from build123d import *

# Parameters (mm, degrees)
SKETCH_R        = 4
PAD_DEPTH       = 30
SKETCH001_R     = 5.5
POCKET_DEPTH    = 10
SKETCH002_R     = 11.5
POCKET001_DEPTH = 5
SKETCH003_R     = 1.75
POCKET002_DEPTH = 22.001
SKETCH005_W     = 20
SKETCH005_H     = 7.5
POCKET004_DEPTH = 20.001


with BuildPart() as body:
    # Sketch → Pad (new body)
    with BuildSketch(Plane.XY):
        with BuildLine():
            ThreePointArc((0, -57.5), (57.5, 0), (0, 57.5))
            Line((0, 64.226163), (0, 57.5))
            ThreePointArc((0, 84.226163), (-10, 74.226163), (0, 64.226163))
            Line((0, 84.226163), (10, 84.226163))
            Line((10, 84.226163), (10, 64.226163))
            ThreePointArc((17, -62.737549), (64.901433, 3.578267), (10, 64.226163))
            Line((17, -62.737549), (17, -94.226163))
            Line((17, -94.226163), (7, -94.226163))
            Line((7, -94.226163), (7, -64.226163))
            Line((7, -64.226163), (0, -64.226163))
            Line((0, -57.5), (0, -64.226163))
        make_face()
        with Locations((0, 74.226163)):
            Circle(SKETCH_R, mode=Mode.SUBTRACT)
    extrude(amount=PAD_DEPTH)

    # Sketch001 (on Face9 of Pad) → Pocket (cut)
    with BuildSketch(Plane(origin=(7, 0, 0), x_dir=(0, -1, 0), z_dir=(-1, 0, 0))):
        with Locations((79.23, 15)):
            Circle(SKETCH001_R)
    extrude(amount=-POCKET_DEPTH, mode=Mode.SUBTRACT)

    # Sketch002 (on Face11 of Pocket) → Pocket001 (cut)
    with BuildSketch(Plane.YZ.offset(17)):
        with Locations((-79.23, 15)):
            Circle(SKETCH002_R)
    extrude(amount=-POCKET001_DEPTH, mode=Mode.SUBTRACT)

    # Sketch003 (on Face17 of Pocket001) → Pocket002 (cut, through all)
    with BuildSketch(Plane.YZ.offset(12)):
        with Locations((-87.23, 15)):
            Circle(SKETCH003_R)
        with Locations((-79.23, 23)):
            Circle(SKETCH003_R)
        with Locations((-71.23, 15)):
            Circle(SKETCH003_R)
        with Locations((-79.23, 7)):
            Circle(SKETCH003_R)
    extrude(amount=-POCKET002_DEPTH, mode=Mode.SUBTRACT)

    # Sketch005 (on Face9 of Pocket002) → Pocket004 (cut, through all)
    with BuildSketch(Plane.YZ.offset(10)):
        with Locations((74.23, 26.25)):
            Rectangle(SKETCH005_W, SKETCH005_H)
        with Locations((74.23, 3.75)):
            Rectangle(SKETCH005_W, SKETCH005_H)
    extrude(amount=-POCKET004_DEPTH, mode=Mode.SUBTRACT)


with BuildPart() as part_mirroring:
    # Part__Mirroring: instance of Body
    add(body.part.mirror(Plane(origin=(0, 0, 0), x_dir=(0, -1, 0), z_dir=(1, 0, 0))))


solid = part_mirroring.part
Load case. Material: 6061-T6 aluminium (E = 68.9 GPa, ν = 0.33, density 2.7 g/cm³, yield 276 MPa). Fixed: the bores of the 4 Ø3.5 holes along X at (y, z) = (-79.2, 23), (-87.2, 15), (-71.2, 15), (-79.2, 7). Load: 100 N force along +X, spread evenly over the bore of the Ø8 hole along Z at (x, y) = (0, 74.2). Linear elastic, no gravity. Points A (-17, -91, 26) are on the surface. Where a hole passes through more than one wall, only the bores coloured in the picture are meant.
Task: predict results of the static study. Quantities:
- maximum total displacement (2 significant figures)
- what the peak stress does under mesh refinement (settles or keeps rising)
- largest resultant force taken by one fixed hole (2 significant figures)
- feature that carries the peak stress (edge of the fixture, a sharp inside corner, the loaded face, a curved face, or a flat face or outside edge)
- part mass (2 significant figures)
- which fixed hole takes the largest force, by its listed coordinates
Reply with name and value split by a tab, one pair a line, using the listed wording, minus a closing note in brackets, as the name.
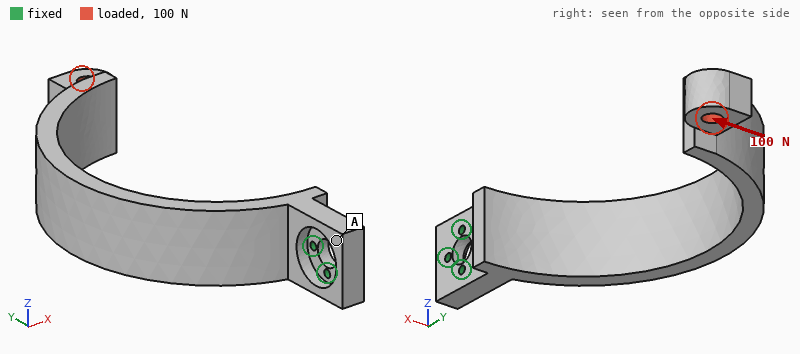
maximum total displacement	2.2 mm
what the peak stress does under mesh refinement	keeps rising
largest resultant force taken by one fixed hole	960 N
feature that carries the peak stress	edge of the fixture
part mass	150 g
which fixed hole takes the largest force, by its listed coordinates	(-71.2, 15)
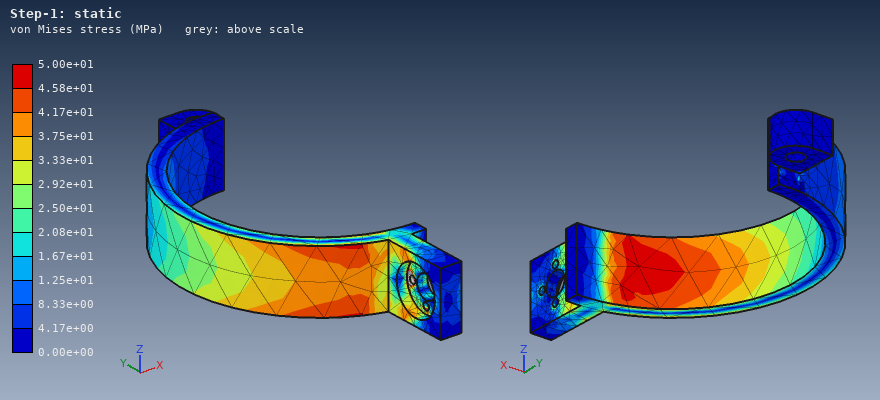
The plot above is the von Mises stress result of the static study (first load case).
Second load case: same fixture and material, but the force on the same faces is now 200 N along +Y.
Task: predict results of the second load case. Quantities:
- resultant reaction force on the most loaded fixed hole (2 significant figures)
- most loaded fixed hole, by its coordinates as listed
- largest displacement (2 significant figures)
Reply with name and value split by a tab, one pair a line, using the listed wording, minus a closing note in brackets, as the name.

resultant reaction force on the most loaded fixed hole	180 N
most loaded fixed hole, by its coordinates as listed	(-71.2, 15)
largest displacement	2.0 mm
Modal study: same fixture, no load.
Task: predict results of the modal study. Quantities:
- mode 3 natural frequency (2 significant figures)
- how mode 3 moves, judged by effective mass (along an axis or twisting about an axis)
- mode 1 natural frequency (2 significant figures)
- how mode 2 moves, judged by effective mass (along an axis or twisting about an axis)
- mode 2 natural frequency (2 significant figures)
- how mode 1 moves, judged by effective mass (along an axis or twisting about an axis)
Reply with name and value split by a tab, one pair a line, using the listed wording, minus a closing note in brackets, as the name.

mode 3 natural frequency	540 Hz
how mode 3 moves, judged by effective mass	along Y
mode 1 natural frequency	170 Hz
how mode 2 moves, judged by effective mass	along Z
mode 2 natural frequency	270 Hz
how mode 1 moves, judged by effective mass	along X
